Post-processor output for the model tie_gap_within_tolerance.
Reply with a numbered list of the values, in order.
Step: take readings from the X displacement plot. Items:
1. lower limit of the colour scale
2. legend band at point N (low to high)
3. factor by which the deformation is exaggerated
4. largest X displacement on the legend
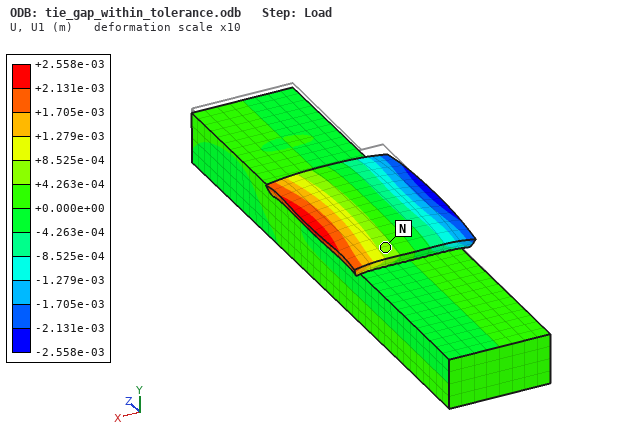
1. -2.558e-03 m
2. +4.263e-04 to +8.525e-04 m
3. 10
4. +2.558e-03 m
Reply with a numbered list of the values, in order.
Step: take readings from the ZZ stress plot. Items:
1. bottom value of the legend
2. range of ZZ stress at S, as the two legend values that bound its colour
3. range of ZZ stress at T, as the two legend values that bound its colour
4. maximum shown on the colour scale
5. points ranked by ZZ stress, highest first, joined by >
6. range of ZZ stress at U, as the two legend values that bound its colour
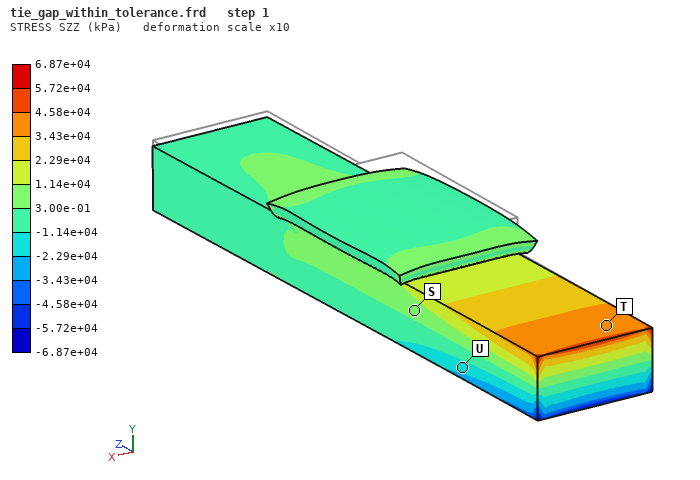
1. -6.87e+04 kPa
2. 3.00e-01 to 1.14e+04 kPa
3. 3.43e+04 to 4.58e+04 kPa
4. 6.87e+04 kPa
5. T > S > U
6. -2.29e+04 to -1.14e+04 kPa
